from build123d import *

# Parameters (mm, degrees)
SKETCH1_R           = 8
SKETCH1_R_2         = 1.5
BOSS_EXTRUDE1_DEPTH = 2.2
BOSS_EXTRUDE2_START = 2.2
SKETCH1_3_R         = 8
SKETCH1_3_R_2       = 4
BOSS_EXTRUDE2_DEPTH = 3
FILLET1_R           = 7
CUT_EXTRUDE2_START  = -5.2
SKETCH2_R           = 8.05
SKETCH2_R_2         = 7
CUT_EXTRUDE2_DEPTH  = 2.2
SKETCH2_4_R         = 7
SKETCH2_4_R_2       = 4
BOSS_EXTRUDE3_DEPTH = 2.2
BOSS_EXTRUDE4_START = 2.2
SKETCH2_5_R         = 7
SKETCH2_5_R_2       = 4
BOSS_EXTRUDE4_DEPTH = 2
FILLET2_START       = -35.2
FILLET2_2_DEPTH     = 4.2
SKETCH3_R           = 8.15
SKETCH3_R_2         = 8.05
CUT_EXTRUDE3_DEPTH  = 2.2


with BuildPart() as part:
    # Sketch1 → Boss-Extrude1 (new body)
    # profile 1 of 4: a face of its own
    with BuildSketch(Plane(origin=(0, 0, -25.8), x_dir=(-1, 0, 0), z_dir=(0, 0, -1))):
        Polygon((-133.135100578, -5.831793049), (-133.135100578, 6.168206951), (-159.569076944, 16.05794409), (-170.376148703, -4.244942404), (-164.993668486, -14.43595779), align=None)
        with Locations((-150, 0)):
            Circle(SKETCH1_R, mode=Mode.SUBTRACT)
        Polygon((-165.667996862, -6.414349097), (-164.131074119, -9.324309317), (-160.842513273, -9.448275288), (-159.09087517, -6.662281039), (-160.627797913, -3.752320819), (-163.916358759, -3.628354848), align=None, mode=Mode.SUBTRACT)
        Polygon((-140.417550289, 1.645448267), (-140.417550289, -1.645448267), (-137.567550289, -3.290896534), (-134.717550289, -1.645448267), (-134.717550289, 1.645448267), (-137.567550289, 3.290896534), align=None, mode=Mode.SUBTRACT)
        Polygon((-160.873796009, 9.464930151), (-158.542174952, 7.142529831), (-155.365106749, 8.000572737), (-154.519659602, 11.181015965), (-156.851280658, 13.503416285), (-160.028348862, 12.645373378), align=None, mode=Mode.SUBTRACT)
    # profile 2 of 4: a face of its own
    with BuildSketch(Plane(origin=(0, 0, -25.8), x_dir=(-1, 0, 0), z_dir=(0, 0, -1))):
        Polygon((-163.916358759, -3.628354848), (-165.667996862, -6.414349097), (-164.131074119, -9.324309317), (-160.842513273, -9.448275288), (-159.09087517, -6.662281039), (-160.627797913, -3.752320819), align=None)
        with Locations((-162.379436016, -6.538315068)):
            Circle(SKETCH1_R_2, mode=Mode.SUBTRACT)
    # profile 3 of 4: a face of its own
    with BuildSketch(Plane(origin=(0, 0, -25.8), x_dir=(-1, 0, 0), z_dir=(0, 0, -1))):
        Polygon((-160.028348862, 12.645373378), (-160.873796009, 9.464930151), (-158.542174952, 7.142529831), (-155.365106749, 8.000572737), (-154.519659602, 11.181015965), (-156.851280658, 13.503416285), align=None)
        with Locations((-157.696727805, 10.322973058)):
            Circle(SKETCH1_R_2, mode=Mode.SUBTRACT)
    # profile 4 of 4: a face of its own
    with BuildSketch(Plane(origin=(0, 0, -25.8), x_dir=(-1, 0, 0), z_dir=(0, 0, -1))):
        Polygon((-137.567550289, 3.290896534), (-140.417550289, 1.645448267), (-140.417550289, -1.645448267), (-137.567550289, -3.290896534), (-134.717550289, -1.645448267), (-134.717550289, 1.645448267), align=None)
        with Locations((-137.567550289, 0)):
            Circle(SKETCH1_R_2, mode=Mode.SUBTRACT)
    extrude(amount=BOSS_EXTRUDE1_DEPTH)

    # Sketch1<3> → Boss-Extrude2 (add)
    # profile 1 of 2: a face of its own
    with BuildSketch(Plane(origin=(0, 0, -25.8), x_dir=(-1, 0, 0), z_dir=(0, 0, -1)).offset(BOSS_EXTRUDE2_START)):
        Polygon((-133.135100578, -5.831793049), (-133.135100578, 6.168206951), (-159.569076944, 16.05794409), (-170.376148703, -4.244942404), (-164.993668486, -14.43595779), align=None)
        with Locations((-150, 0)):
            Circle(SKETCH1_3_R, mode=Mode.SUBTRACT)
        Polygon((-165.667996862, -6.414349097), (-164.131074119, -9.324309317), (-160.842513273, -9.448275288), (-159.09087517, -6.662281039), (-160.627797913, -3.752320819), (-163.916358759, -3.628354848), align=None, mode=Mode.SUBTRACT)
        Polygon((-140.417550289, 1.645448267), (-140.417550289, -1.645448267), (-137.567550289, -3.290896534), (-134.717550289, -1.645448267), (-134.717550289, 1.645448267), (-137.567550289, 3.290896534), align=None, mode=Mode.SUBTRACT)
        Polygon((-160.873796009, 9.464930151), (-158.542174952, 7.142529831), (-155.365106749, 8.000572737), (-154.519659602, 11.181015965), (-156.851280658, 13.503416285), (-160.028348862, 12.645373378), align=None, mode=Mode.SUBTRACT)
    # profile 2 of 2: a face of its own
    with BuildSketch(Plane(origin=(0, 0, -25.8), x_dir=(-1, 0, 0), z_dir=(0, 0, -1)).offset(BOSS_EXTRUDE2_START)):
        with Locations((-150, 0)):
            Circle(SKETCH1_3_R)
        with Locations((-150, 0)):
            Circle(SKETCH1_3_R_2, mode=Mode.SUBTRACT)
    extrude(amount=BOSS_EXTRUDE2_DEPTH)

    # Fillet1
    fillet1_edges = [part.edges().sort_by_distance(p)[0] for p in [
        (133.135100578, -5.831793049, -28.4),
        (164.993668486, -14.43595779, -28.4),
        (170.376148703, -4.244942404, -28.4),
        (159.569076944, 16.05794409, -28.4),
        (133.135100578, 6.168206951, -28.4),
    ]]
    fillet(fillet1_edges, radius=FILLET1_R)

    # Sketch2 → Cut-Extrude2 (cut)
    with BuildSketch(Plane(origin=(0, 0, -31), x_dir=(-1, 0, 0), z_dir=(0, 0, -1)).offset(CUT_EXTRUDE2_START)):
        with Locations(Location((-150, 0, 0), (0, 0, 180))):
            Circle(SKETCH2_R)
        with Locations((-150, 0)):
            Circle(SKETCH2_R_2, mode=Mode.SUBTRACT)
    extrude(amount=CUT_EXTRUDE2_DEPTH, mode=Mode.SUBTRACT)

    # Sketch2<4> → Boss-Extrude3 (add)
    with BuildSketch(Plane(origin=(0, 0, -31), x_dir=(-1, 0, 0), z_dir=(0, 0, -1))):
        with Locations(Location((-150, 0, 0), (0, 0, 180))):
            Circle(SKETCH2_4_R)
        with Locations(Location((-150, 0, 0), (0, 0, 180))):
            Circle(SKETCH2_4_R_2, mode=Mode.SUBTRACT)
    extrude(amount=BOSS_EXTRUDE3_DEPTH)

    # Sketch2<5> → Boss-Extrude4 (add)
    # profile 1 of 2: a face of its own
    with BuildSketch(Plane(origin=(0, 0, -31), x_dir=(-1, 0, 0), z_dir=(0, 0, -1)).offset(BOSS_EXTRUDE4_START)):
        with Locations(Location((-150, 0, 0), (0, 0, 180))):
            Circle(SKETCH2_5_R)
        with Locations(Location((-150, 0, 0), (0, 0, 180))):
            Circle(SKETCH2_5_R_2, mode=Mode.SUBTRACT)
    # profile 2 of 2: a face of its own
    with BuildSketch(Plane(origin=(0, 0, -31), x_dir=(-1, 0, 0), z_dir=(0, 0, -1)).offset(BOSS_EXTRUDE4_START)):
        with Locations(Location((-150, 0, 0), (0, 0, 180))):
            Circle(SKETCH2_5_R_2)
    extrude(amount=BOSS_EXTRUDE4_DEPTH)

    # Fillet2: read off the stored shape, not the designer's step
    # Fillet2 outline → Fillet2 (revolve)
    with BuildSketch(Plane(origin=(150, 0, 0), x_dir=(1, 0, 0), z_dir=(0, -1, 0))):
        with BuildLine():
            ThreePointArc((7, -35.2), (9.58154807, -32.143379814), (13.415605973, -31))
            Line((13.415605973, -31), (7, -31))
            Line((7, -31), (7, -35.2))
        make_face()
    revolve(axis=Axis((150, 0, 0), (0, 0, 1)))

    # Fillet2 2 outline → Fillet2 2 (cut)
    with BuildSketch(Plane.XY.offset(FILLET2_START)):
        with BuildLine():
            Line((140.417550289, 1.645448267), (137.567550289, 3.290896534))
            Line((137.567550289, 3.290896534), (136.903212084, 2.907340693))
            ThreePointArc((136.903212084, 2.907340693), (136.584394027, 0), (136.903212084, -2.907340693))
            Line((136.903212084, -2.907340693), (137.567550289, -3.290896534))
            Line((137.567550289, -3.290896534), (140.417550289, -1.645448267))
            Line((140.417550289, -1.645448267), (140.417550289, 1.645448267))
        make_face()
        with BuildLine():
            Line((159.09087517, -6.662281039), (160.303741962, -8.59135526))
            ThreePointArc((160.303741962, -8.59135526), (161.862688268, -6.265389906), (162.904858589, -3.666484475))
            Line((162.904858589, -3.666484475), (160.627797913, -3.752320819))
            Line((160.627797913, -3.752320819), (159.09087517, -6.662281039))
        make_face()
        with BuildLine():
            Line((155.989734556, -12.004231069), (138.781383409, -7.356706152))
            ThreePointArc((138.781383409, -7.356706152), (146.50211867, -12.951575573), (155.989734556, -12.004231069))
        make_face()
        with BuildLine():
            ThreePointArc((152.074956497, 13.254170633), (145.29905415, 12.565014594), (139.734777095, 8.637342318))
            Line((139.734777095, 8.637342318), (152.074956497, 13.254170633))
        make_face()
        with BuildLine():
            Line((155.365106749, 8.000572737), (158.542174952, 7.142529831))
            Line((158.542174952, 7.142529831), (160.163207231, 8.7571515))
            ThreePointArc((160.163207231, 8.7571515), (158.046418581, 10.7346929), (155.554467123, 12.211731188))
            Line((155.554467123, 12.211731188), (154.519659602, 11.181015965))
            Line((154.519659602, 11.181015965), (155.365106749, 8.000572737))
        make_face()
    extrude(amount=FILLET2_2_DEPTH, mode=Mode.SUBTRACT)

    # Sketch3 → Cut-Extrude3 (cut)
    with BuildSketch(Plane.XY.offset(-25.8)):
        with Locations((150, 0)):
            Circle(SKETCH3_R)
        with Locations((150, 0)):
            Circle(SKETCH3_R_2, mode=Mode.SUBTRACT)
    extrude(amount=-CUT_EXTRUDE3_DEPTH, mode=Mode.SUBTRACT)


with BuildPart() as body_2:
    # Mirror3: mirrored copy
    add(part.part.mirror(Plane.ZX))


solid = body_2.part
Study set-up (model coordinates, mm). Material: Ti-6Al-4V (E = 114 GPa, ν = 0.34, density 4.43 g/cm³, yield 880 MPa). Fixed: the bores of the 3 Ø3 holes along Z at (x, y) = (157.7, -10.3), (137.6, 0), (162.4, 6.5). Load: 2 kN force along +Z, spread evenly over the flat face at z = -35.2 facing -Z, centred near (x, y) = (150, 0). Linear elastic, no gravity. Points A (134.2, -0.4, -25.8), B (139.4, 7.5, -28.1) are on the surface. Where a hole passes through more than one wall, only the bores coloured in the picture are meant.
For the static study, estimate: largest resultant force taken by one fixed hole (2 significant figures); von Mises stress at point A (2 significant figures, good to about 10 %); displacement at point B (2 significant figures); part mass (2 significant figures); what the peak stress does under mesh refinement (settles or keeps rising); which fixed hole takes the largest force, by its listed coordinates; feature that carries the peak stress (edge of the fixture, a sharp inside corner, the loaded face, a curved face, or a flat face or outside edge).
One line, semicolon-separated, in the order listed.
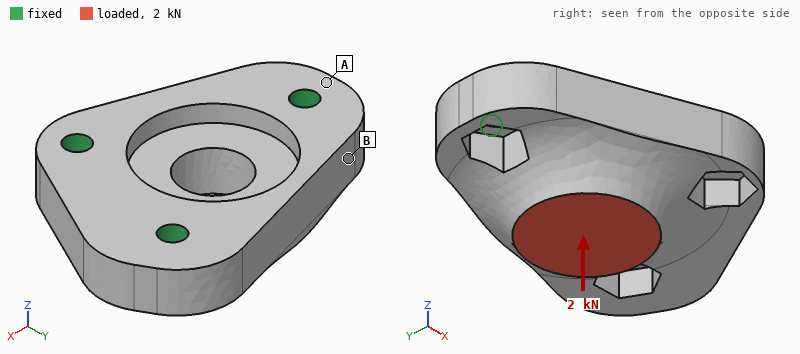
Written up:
1.1 kN; 34 MPa; 5.6 µm; 16 g; keeps rising; (137.6, 0); edge of the fixture
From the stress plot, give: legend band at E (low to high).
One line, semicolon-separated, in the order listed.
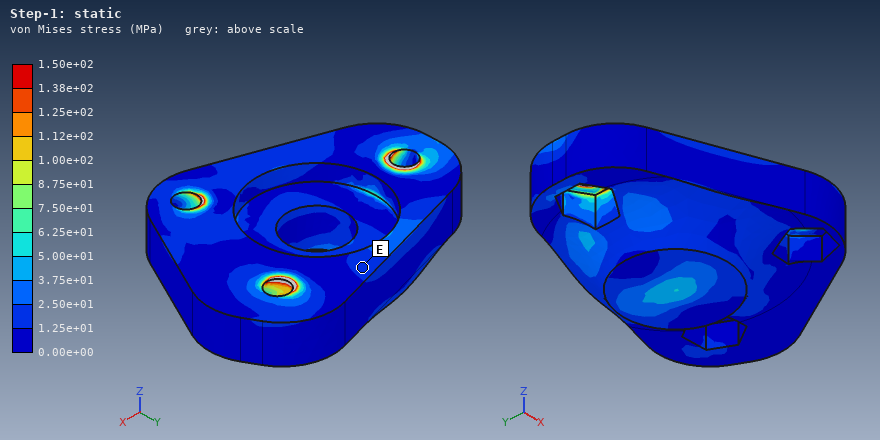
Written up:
1.25e+01 to 2.50e+01 MPa
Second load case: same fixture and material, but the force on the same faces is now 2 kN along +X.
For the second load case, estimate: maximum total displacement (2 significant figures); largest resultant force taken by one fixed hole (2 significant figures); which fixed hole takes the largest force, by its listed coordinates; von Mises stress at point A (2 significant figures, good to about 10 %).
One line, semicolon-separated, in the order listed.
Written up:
5.8 µm; 1.1 kN; (137.6, 0); 41 MPa
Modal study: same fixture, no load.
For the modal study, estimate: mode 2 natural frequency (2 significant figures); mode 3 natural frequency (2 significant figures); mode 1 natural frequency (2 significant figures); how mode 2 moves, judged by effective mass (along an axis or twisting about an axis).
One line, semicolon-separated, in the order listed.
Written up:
31 kHz; 36 kHz; 25 kHz; along Z
